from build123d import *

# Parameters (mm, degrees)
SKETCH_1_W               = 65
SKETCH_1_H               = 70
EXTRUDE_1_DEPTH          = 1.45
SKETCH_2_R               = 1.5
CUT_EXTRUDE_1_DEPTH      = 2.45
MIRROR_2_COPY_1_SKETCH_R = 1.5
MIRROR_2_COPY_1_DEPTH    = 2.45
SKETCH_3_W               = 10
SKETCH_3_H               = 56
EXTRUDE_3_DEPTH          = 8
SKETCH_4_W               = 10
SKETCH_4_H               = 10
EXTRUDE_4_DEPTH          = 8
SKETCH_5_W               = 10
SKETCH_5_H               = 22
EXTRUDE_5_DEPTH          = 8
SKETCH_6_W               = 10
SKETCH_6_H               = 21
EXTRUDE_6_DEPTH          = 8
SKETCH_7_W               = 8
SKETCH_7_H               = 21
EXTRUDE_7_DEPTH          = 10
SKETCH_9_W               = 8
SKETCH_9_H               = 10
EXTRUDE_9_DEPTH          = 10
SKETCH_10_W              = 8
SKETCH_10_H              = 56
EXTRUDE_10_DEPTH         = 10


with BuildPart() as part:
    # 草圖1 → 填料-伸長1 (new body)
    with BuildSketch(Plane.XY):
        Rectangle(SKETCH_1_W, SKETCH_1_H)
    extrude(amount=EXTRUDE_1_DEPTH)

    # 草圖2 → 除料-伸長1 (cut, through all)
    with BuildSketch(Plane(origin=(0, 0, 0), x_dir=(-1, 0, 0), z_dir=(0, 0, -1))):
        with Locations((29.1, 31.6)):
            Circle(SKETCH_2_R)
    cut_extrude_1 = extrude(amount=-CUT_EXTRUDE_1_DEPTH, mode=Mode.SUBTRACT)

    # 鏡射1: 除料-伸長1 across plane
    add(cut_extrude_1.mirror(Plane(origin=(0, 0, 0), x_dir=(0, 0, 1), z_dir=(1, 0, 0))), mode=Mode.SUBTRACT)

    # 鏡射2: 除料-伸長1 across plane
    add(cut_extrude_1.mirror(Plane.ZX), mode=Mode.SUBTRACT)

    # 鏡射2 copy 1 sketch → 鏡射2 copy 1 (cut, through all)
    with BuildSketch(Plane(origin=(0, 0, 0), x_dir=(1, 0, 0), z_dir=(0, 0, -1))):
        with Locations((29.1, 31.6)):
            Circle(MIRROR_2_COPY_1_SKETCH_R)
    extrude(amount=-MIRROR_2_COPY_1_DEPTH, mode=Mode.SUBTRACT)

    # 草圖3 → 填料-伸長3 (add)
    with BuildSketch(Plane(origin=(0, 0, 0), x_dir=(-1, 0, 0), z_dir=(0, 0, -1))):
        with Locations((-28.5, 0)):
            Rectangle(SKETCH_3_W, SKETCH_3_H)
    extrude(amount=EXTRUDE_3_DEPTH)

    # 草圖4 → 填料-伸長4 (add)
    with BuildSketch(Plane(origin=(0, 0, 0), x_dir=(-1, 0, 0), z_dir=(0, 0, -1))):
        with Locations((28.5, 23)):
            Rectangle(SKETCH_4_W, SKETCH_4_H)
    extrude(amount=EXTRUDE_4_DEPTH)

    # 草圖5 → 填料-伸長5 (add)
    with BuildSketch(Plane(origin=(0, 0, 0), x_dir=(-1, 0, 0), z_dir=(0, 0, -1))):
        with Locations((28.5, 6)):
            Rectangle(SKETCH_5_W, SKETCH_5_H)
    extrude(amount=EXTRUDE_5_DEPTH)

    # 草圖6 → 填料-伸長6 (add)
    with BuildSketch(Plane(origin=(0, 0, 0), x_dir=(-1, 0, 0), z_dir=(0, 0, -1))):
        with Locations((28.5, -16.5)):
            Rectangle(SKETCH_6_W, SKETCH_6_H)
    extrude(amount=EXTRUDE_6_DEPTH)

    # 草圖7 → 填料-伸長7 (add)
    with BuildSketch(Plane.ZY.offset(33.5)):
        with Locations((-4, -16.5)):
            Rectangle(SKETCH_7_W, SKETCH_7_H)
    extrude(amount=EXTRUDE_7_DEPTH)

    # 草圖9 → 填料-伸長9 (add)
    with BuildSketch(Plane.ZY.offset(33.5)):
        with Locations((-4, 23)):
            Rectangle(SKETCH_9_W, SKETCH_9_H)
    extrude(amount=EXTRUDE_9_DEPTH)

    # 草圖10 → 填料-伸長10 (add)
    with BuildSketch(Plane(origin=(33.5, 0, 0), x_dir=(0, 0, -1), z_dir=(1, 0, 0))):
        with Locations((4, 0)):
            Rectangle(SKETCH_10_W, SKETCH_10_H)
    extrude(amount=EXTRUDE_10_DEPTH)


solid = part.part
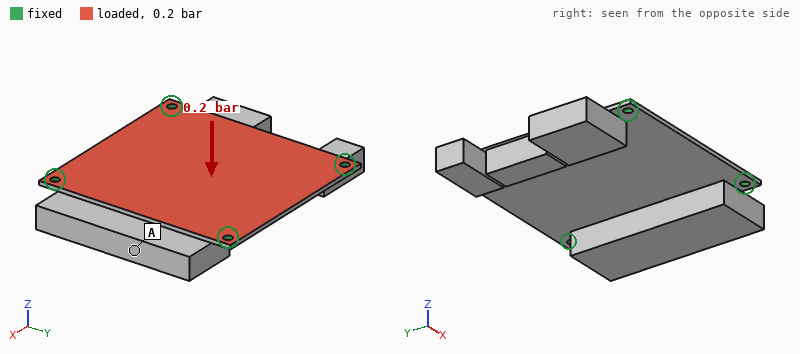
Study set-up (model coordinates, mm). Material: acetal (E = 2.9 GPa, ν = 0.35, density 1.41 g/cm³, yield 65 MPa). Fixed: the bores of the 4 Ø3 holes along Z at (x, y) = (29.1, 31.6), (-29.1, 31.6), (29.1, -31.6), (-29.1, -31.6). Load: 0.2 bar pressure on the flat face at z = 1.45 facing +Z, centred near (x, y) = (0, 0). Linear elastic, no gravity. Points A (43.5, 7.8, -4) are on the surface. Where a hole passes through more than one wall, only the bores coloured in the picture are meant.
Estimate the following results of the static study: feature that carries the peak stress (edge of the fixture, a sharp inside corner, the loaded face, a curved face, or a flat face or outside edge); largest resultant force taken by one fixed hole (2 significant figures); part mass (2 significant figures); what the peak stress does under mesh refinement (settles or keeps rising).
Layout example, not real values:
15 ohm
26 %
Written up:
edge of the fixture
31 N
31 g
keeps rising
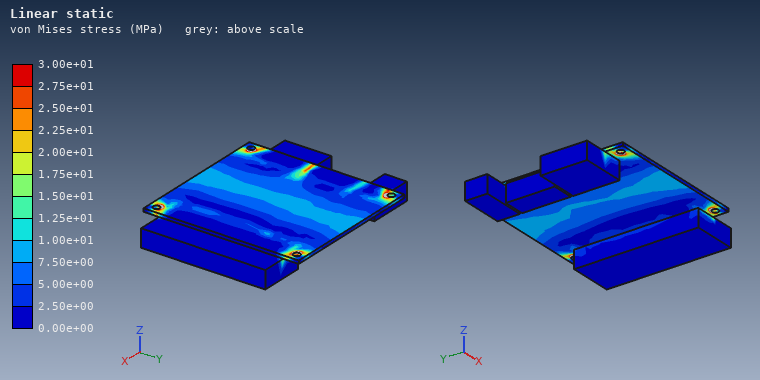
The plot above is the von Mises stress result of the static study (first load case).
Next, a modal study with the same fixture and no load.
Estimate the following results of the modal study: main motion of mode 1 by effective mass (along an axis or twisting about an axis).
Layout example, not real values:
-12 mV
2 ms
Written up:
along Z
